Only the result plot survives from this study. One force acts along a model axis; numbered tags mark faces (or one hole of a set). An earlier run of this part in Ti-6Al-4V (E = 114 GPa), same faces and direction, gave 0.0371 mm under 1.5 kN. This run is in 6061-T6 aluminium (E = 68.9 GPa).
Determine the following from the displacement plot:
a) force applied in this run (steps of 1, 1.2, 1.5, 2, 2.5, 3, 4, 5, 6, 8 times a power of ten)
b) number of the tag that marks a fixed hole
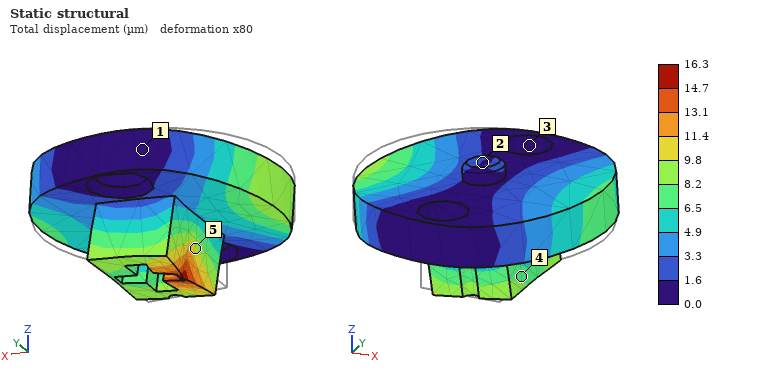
400 N
3
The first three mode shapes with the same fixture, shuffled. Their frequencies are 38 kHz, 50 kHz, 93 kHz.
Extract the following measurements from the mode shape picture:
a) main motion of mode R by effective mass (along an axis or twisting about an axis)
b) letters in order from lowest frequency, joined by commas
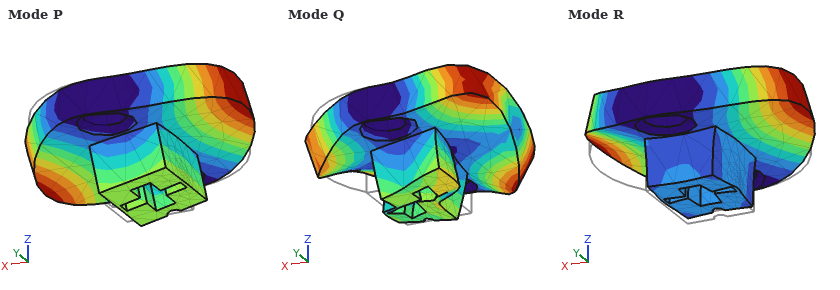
along Z
P, R, Q
